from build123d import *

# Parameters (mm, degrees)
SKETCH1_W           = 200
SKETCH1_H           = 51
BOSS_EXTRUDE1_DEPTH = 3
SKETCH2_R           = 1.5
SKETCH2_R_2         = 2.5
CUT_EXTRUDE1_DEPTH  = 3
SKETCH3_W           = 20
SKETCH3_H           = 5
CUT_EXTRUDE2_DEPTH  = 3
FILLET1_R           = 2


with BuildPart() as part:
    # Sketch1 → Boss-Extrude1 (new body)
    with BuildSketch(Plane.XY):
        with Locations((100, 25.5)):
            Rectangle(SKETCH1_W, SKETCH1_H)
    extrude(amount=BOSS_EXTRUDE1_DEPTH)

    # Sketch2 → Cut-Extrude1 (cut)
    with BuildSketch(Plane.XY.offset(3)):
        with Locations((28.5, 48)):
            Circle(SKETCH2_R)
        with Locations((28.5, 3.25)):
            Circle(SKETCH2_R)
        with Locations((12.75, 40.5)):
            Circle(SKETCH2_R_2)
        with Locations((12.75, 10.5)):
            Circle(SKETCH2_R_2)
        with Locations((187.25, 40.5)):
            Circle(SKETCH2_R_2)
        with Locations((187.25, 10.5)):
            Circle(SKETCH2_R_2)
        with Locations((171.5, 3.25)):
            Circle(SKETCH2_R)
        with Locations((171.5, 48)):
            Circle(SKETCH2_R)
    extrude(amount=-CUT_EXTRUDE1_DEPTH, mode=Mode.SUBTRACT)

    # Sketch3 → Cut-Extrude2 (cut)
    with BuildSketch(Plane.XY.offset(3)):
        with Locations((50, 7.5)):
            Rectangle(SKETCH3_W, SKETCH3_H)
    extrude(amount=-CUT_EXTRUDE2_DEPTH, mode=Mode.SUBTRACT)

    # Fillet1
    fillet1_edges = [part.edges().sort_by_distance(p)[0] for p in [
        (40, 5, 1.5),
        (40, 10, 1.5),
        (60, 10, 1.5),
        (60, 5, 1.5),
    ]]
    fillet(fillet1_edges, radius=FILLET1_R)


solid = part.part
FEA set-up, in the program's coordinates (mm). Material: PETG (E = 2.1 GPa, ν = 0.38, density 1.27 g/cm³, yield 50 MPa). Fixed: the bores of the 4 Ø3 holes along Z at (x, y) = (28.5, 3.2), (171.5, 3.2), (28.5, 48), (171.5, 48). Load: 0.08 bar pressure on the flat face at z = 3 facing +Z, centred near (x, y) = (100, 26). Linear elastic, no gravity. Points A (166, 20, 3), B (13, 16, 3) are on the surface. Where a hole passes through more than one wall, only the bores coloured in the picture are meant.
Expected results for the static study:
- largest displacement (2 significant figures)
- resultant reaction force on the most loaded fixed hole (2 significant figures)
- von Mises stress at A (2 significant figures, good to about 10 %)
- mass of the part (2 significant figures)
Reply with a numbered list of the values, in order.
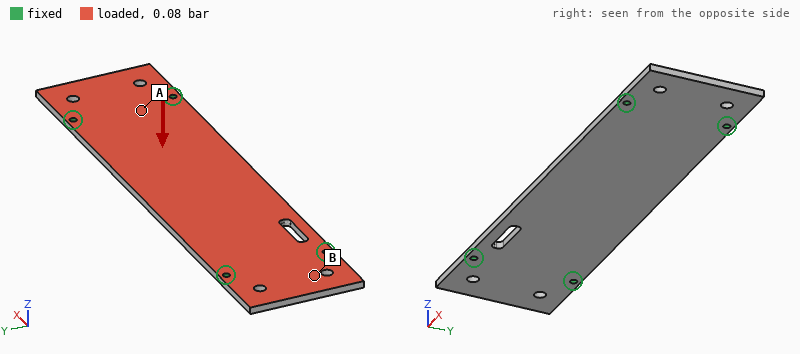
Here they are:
1. 2.2 mm
2. 20 N
3. 4.4 MPa
4. 38 g
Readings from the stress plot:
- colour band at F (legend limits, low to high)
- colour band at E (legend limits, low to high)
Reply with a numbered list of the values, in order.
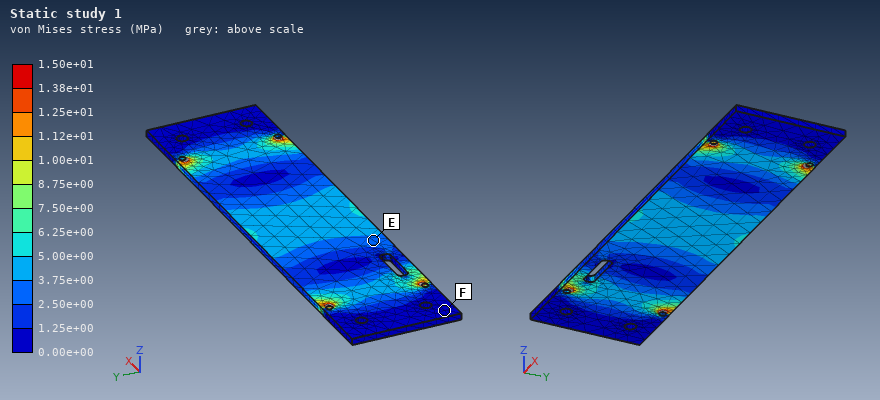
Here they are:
1. 0.00e+00 to 1.25e+00 MPa
2. 2.50e+00 to 3.75e+00 MPa
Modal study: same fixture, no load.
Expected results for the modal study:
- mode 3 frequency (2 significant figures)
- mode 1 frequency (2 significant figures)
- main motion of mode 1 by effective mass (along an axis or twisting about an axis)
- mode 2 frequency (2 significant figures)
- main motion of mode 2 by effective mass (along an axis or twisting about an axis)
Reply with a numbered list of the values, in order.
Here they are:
1. 480 Hz
2. 180 Hz
3. along Z
4. 390 Hz
5. twisting about X
